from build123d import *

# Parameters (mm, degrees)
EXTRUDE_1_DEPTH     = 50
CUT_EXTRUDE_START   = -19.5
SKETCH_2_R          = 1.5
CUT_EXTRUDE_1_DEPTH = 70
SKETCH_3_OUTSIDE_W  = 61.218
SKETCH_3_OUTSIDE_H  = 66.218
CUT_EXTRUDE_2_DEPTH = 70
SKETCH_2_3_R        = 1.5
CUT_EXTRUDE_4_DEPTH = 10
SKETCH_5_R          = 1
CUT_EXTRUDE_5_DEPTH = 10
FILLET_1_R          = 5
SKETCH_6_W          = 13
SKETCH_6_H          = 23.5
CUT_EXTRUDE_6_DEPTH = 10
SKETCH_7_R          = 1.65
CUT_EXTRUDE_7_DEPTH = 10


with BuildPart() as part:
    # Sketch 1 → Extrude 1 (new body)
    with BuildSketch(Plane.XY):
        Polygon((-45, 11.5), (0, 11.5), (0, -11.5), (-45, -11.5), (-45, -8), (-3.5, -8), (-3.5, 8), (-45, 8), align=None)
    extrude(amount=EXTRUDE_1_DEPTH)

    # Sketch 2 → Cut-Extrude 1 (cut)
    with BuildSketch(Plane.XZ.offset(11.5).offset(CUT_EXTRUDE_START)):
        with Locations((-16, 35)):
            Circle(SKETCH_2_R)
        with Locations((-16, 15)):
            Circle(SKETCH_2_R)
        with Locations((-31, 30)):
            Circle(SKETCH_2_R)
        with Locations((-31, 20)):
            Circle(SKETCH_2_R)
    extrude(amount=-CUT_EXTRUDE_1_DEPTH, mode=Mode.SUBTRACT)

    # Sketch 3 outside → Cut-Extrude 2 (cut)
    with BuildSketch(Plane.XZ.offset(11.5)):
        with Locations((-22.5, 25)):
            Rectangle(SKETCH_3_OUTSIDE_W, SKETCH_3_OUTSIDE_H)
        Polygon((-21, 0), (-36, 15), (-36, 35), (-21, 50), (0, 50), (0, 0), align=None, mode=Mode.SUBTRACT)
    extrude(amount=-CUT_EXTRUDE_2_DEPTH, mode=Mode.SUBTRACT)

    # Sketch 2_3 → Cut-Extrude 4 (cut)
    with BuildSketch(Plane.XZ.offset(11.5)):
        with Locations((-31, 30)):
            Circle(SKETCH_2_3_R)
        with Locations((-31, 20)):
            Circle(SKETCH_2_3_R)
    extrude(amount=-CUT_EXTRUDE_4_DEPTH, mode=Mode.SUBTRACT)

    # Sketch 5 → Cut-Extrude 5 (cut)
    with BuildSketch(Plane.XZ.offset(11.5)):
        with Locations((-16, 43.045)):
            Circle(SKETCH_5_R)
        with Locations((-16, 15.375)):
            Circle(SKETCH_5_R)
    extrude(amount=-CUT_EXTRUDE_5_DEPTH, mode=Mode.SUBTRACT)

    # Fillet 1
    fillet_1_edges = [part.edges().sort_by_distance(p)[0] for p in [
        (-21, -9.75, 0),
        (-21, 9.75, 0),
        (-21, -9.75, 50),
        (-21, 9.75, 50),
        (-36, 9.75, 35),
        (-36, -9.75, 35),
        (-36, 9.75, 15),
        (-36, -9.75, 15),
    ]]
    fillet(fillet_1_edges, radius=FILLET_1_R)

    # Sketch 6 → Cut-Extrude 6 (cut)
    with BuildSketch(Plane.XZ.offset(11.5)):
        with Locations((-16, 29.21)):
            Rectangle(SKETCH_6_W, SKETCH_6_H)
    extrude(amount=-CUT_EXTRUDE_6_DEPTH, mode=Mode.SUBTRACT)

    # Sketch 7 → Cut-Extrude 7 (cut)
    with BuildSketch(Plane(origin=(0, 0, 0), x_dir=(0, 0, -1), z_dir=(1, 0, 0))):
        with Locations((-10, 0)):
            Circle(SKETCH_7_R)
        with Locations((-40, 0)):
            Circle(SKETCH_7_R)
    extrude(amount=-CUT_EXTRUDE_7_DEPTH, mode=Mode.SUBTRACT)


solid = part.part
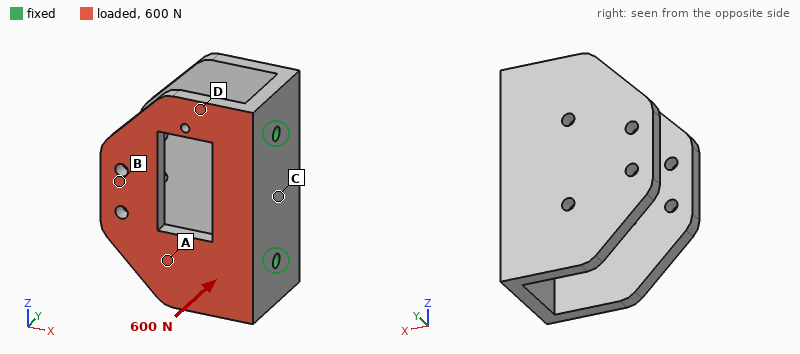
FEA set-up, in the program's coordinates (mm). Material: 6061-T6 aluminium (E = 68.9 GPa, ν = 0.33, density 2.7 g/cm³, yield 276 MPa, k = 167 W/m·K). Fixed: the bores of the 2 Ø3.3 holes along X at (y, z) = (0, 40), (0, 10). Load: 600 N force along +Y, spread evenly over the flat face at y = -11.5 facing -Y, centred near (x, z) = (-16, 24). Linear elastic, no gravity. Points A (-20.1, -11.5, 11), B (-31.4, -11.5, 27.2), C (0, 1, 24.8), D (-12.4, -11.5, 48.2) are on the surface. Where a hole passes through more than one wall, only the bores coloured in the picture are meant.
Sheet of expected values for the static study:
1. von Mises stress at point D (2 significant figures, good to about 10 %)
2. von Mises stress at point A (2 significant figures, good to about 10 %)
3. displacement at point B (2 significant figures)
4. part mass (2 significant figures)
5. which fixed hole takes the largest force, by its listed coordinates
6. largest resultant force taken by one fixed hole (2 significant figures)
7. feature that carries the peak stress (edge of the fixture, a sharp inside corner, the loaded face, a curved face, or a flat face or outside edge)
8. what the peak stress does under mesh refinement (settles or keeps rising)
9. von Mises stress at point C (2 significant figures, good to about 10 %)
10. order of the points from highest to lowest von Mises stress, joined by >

79 MPa
42 MPa
0.49 mm
34 g
(0, 10)
320 N
edge of the fixture
keeps rising
28 MPa
D > A > C > B
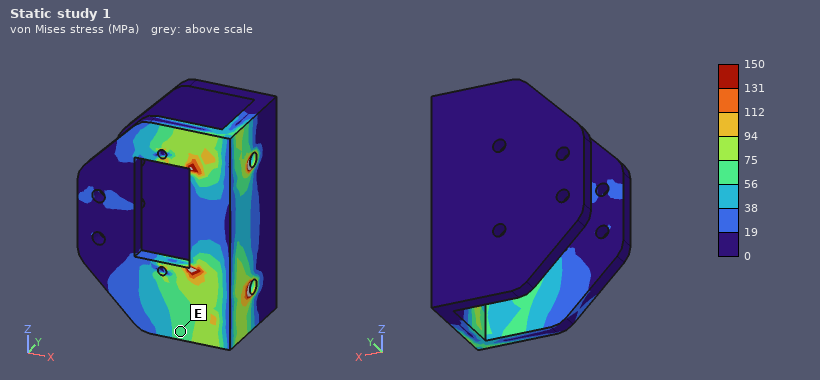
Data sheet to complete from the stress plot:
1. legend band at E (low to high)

56 to 75 MPa
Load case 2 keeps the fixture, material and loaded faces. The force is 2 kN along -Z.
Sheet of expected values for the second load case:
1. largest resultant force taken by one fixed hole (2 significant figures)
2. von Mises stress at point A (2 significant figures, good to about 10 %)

1.5 kN
25 MPa
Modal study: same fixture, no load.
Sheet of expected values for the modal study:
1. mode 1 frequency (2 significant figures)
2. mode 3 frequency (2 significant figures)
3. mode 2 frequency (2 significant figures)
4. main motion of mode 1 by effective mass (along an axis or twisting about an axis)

1800 Hz
4300 Hz
2100 Hz
along Y
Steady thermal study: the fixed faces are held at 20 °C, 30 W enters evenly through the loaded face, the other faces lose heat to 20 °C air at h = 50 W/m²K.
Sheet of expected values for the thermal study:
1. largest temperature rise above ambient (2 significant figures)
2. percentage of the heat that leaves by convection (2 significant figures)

38 K
12 %
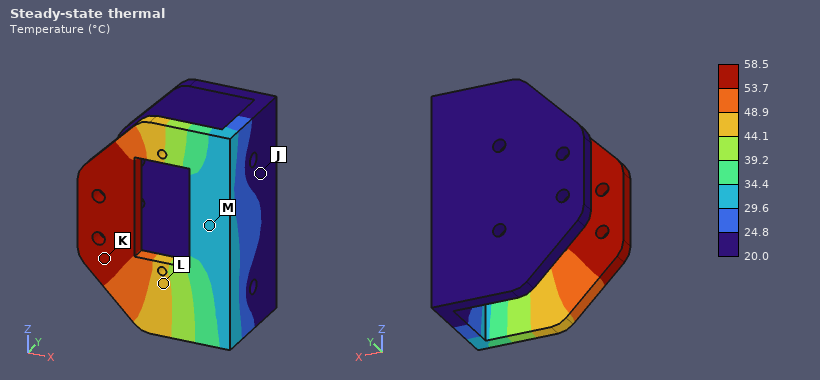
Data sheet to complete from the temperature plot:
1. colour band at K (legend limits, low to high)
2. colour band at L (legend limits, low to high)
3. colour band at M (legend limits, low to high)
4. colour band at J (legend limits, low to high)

53.7 to 58.5 °C
44.1 to 48.9 °C
29.6 to 34.4 °C
20.0 to 24.8 °C
